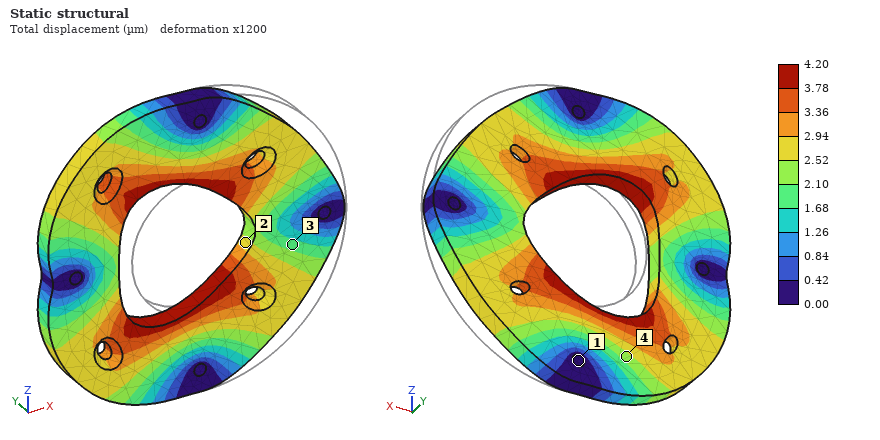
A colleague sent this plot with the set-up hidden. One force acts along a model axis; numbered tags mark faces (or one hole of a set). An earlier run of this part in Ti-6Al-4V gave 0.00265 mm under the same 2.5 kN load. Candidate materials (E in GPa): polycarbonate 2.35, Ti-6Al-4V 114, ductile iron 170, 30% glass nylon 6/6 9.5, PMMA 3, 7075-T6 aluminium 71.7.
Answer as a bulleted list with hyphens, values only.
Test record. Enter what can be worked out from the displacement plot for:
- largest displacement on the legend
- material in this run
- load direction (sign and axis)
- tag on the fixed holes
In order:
- 4.20 µm
- 7075-T6 aluminium
- -X
- 1
